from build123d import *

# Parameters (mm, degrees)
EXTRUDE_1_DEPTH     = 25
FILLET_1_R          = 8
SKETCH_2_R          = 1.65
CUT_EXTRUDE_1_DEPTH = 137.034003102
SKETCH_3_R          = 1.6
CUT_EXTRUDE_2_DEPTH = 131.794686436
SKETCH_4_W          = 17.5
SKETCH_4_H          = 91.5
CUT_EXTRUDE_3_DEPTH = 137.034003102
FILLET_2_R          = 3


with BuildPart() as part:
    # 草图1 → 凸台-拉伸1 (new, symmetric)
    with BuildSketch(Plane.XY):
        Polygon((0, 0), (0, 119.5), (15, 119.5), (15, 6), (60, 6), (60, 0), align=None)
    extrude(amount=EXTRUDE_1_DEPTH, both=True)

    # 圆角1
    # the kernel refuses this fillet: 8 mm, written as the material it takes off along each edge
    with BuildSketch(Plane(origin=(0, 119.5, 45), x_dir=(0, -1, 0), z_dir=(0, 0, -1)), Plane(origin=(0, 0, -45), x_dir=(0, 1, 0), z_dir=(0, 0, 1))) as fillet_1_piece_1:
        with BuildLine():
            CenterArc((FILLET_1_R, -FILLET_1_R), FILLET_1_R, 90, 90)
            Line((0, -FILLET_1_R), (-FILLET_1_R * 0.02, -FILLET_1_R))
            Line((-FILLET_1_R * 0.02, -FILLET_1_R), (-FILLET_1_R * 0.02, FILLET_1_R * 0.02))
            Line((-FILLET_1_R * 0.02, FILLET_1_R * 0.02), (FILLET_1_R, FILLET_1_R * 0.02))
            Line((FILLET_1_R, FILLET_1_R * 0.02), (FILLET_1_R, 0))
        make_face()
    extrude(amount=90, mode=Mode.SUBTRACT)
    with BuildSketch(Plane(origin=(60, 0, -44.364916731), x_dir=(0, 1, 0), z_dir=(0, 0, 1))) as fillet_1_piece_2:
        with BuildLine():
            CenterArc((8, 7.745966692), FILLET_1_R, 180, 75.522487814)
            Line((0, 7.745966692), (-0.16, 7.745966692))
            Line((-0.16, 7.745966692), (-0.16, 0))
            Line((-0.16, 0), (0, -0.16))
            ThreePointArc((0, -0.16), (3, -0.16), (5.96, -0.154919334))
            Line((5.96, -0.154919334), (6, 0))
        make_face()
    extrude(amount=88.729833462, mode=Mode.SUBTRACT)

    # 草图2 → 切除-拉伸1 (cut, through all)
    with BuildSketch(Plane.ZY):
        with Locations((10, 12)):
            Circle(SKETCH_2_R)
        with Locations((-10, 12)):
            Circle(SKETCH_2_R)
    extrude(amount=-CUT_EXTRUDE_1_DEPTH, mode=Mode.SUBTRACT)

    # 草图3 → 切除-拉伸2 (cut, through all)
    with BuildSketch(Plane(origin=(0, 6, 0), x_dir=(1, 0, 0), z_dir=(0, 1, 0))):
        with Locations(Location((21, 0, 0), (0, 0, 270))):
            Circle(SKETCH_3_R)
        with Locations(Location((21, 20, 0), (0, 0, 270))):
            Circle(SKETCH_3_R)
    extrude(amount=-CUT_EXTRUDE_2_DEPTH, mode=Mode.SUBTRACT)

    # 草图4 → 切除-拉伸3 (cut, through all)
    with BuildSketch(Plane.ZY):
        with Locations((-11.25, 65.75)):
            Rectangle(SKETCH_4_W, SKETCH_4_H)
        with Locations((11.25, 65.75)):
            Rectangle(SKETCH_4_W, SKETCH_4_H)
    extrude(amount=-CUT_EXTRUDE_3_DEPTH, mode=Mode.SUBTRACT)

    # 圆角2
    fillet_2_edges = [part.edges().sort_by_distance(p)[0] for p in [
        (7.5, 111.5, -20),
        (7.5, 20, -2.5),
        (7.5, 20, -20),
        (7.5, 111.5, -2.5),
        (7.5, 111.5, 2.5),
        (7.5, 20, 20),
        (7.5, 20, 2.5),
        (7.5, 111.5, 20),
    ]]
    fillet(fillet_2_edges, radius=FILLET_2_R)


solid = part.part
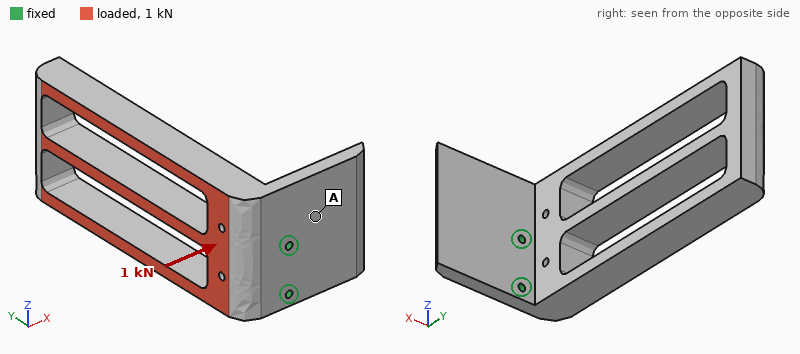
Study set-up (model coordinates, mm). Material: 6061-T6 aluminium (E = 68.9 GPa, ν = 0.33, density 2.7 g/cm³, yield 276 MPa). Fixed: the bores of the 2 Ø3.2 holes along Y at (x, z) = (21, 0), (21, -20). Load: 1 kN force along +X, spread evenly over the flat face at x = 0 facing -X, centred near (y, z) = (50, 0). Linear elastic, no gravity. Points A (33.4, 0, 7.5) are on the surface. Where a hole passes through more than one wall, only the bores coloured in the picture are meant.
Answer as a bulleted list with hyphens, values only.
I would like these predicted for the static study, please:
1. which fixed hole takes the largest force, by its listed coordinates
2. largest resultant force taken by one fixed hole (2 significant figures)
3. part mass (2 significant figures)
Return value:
- (21, 0)
- 970 N
- 140 g
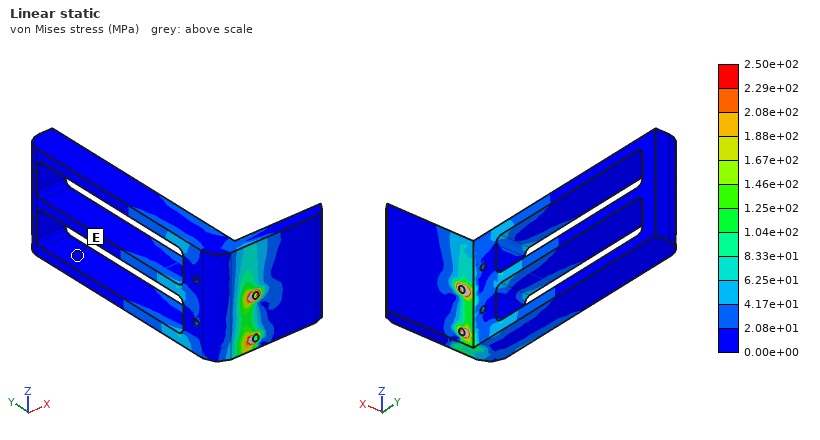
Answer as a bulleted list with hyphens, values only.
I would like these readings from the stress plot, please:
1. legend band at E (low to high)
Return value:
- 0.00e+00 to 2.08e+01 MPa
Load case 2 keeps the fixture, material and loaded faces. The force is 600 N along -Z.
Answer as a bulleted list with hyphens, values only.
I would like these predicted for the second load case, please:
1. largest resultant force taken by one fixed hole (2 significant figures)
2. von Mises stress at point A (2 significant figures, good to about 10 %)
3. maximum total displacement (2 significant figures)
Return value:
- 1.4 kN
- 11 MPa
- 0.58 mm
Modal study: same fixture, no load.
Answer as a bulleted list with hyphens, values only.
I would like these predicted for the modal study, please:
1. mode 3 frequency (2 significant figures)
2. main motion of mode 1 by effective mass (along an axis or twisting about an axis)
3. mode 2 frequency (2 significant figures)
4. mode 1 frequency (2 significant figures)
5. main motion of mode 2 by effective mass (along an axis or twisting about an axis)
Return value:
- 1600 Hz
- along X
- 520 Hz
- 450 Hz
- along Z
